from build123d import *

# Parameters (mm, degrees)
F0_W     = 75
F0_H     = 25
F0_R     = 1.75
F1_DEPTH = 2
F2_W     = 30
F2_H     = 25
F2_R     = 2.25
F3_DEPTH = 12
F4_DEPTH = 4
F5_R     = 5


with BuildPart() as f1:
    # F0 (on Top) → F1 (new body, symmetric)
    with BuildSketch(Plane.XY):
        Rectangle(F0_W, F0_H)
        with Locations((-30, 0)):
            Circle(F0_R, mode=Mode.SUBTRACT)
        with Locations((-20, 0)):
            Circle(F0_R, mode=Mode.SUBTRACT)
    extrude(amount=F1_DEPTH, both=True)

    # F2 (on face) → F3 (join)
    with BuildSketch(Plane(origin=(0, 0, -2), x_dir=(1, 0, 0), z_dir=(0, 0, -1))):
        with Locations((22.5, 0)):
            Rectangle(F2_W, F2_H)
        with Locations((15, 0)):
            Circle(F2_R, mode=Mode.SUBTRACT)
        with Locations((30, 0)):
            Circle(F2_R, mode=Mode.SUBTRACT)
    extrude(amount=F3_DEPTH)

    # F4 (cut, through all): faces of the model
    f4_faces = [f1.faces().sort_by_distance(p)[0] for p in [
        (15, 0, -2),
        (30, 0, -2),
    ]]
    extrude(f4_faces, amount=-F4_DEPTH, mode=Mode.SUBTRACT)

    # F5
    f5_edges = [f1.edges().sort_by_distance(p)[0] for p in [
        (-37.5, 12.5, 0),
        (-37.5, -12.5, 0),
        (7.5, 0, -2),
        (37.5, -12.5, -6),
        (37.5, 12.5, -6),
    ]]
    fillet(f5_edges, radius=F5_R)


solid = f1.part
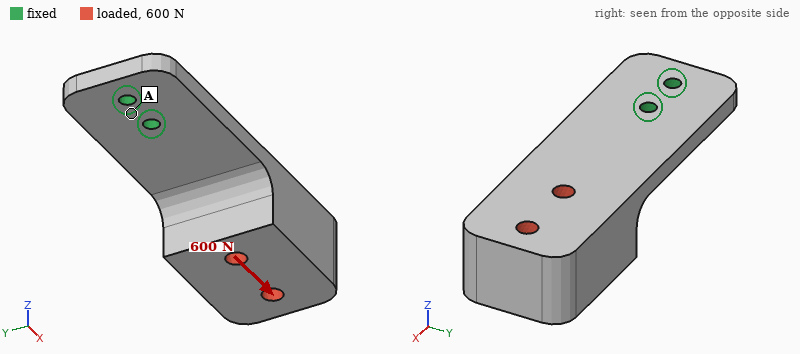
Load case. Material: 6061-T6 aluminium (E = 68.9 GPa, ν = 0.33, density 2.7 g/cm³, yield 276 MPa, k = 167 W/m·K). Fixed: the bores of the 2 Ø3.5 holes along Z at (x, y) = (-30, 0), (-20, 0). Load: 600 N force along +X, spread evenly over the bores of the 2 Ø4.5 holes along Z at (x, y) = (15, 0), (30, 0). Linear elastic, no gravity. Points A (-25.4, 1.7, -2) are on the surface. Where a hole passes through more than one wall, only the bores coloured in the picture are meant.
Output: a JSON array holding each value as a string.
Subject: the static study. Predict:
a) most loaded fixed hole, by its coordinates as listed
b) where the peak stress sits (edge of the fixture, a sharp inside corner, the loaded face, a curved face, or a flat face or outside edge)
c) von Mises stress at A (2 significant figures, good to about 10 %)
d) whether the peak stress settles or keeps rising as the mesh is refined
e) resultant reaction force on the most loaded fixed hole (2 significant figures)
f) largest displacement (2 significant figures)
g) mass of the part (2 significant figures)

["(-20, 0)", "edge of the fixture", "12 MPa", "keeps rising", "460 N", "0.48 mm", "43 g"]
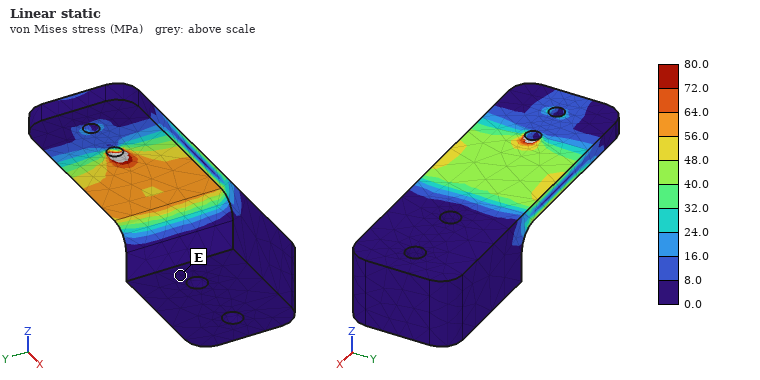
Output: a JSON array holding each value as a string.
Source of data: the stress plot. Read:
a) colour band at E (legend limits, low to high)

["0.0 to 8.0 MPa"]
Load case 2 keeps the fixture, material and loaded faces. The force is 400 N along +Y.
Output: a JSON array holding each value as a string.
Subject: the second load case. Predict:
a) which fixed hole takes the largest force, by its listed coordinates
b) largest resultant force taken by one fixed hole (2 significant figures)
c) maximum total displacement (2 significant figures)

["(-20, 0)", "1.6 kN", "0.16 mm"]
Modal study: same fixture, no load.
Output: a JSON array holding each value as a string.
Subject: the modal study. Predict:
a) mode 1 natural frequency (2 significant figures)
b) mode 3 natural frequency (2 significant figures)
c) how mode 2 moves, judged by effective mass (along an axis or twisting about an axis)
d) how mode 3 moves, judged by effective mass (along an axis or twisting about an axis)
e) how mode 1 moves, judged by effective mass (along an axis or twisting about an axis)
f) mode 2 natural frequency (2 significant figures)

["520 Hz", "2900 Hz", "along Y", "along Y", "along Z", "1700 Hz"]
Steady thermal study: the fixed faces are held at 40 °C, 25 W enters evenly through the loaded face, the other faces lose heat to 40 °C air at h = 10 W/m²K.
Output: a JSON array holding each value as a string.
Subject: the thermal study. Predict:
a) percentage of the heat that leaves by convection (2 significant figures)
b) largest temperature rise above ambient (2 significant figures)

["7.1 %", "50 K"]
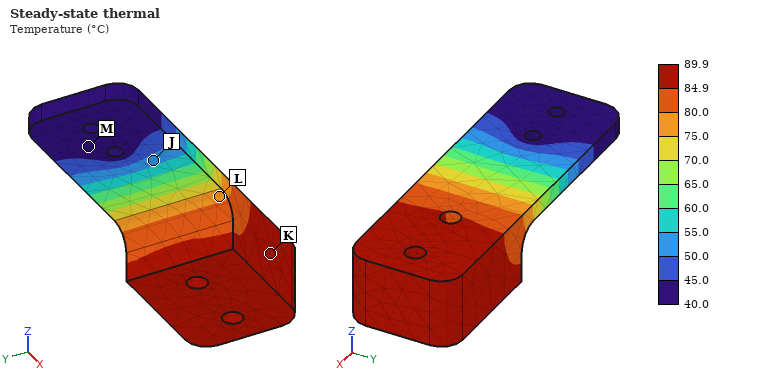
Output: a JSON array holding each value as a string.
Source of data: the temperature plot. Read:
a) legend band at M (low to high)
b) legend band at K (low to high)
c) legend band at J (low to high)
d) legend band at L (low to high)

["40.0 to 45.0 °C", "84.9 to 89.9 °C", "50.0 to 55.0 °C", "75.0 to 80.0 °C"]
